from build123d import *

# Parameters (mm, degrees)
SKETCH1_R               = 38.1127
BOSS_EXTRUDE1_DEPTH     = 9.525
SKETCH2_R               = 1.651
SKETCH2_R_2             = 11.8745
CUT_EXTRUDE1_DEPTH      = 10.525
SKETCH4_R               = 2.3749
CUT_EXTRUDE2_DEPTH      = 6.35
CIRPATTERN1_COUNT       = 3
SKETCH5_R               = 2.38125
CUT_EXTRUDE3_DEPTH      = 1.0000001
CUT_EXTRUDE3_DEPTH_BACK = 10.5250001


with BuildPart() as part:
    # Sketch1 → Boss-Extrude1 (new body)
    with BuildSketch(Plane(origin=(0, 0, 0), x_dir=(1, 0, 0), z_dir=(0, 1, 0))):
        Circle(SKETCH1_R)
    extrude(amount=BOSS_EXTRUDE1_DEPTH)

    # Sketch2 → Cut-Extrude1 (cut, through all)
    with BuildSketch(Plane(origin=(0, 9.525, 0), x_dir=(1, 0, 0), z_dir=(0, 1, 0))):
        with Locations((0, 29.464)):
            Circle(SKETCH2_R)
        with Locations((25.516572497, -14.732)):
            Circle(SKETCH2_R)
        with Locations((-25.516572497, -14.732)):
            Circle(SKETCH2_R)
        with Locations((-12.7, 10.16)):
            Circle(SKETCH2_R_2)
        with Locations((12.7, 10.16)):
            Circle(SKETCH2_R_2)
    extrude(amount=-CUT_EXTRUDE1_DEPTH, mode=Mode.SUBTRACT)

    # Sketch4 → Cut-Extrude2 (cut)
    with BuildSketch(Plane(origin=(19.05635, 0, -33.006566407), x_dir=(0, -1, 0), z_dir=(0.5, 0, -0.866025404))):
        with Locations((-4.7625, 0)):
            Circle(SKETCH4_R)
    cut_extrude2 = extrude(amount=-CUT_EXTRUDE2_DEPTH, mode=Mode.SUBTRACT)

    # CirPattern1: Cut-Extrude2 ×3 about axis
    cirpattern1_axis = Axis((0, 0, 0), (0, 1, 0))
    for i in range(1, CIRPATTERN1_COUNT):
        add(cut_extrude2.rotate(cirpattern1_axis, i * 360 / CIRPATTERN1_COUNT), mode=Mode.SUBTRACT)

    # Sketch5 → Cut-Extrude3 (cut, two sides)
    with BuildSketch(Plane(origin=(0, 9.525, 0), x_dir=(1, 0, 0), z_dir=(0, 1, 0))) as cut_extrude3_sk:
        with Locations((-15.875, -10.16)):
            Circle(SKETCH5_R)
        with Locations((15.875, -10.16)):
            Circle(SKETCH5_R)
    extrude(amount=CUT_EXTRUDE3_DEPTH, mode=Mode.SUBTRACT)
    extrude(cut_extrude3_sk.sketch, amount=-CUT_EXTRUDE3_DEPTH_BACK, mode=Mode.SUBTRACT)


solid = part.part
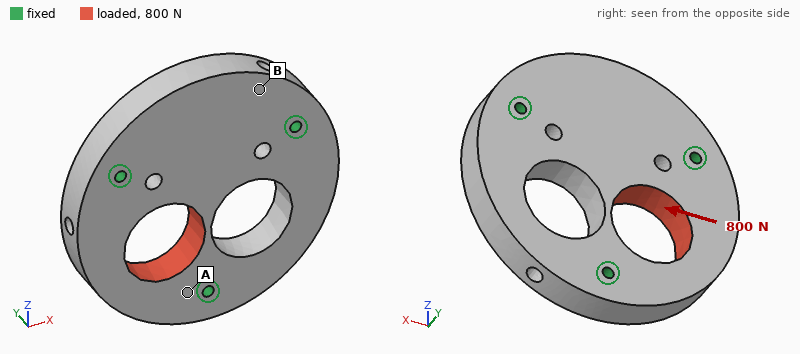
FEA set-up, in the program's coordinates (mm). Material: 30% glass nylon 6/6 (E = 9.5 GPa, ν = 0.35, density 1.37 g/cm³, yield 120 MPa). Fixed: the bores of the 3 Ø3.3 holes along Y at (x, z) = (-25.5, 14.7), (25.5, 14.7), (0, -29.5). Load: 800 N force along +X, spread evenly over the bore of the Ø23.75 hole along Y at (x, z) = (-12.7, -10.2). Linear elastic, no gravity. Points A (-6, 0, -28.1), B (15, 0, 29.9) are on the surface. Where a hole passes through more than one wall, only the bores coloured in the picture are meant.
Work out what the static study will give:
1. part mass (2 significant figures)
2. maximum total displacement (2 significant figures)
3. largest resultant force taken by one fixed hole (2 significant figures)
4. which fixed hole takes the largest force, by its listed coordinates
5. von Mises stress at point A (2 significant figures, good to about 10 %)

47 g
17 µm
420 N
(0, -29.5)
3.9 MPa
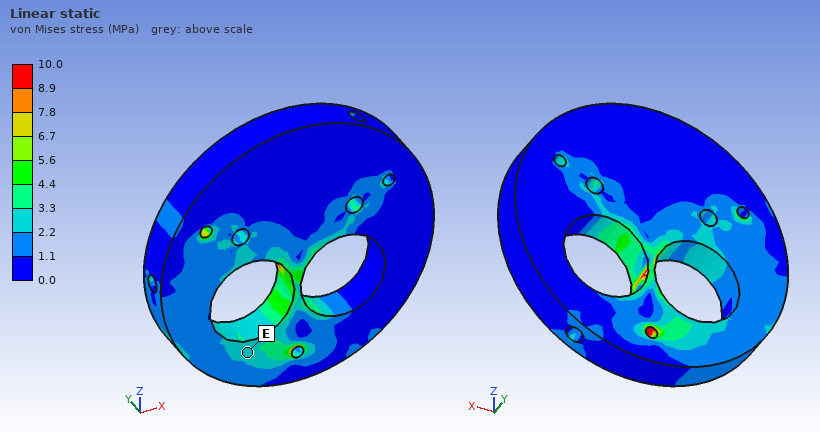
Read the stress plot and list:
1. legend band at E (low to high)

2.2 to 3.3 MPa
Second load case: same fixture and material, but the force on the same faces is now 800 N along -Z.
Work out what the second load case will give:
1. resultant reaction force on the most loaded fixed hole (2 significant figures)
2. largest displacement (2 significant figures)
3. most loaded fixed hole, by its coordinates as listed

450 N
11 µm
(-25.5, 14.7)
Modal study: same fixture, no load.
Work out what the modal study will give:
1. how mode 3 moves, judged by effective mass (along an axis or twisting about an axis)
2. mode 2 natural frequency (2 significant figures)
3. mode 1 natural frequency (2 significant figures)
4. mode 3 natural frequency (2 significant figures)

along Y
4600 Hz
4500 Hz
5400 Hz
